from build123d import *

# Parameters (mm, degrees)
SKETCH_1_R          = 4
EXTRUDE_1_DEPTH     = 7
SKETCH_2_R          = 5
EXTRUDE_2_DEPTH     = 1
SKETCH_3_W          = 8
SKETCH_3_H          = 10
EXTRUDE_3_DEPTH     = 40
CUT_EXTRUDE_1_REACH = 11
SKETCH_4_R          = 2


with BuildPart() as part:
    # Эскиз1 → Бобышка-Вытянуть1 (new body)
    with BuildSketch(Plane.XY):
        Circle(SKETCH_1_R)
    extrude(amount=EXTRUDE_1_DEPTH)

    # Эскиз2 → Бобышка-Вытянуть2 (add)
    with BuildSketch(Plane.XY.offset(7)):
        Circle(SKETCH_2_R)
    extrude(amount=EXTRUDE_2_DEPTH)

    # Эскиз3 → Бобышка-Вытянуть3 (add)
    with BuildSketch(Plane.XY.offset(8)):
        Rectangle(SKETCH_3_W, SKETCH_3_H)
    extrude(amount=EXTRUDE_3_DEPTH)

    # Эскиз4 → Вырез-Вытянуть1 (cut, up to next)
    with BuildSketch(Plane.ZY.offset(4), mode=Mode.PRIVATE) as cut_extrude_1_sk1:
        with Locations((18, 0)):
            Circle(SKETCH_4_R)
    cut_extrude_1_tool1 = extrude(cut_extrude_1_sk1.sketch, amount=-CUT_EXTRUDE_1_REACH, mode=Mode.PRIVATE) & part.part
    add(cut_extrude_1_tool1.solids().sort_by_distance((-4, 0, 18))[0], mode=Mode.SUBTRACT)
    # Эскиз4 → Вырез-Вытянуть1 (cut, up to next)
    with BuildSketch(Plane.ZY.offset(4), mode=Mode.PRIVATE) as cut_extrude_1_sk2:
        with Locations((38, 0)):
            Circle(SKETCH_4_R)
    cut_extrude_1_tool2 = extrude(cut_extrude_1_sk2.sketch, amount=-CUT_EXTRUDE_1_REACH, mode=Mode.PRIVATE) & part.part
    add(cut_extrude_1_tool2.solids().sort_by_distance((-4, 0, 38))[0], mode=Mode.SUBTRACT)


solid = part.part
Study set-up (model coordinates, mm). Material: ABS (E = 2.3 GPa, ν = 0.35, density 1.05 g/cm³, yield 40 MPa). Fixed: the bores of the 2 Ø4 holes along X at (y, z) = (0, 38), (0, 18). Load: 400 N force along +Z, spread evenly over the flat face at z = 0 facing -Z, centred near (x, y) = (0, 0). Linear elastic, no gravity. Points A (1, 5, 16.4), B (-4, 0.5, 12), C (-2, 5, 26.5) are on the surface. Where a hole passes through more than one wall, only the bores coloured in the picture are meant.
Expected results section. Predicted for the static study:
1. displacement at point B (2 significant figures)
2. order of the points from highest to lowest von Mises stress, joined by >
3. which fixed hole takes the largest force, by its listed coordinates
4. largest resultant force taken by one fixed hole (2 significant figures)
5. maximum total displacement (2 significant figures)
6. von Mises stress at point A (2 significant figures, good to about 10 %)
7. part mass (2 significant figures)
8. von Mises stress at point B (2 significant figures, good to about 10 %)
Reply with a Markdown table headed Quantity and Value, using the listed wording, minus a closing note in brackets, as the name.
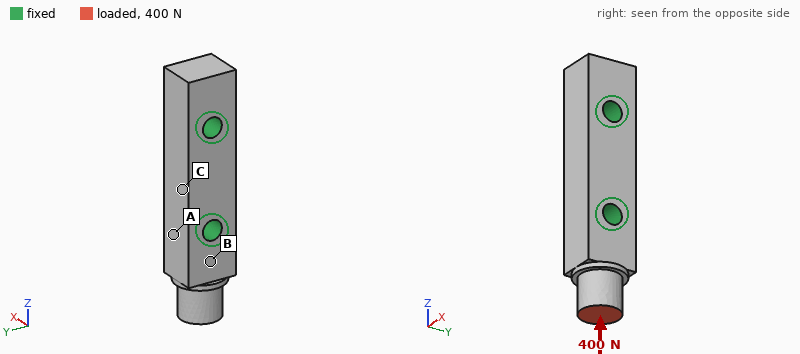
| Quantity | Value |
|---|---|
| displacement at point B | 13 µm |
| order of the points from highest to lowest von Mises stress, joined by > | B > A > C |
| which fixed hole takes the largest force, by its listed coordinates | (0, 18) |
| largest resultant force taken by one fixed hole | 380 N |
| maximum total displacement | 50 µm |
| von Mises stress at point A | 2.5 MPa |
| part mass | 3.6 g |
| von Mises stress at point B | 6.8 MPa |
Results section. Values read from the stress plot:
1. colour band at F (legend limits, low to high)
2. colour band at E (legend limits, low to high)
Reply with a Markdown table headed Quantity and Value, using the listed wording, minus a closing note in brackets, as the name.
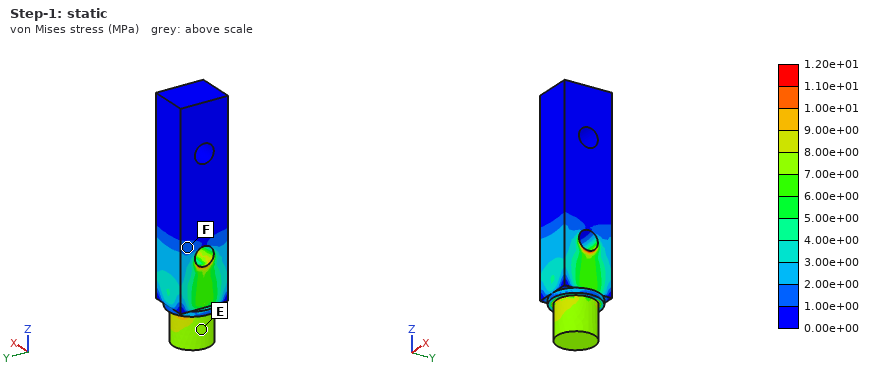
| Quantity | Value |
|---|---|
| colour band at F | 1.00e+00 to 2.00e+00 MPa |
| colour band at E | 7.00e+00 to 8.00e+00 MPa |
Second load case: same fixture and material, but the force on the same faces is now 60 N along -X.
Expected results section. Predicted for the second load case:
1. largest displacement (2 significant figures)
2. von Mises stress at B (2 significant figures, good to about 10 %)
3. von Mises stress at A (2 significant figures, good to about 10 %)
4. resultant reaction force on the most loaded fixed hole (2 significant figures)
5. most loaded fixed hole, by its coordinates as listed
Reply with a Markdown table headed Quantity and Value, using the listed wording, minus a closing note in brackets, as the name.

| Quantity | Value |
|---|---|
| largest displacement | 0.15 mm |
| von Mises stress at B | 8.0 MPa |
| von Mises stress at A | 1.9 MPa |
| resultant reaction force on the most loaded fixed hole | 65 N |
| most loaded fixed hole, by its coordinates as listed | (0, 18) |
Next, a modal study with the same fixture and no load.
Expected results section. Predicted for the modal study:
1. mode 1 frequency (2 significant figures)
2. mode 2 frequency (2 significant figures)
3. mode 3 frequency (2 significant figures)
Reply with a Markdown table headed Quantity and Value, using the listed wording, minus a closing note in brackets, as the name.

| Quantity | Value |
|---|---|
| mode 1 frequency | 6500 Hz |
| mode 2 frequency | 6600 Hz |
| mode 3 frequency | 14 kHz |
